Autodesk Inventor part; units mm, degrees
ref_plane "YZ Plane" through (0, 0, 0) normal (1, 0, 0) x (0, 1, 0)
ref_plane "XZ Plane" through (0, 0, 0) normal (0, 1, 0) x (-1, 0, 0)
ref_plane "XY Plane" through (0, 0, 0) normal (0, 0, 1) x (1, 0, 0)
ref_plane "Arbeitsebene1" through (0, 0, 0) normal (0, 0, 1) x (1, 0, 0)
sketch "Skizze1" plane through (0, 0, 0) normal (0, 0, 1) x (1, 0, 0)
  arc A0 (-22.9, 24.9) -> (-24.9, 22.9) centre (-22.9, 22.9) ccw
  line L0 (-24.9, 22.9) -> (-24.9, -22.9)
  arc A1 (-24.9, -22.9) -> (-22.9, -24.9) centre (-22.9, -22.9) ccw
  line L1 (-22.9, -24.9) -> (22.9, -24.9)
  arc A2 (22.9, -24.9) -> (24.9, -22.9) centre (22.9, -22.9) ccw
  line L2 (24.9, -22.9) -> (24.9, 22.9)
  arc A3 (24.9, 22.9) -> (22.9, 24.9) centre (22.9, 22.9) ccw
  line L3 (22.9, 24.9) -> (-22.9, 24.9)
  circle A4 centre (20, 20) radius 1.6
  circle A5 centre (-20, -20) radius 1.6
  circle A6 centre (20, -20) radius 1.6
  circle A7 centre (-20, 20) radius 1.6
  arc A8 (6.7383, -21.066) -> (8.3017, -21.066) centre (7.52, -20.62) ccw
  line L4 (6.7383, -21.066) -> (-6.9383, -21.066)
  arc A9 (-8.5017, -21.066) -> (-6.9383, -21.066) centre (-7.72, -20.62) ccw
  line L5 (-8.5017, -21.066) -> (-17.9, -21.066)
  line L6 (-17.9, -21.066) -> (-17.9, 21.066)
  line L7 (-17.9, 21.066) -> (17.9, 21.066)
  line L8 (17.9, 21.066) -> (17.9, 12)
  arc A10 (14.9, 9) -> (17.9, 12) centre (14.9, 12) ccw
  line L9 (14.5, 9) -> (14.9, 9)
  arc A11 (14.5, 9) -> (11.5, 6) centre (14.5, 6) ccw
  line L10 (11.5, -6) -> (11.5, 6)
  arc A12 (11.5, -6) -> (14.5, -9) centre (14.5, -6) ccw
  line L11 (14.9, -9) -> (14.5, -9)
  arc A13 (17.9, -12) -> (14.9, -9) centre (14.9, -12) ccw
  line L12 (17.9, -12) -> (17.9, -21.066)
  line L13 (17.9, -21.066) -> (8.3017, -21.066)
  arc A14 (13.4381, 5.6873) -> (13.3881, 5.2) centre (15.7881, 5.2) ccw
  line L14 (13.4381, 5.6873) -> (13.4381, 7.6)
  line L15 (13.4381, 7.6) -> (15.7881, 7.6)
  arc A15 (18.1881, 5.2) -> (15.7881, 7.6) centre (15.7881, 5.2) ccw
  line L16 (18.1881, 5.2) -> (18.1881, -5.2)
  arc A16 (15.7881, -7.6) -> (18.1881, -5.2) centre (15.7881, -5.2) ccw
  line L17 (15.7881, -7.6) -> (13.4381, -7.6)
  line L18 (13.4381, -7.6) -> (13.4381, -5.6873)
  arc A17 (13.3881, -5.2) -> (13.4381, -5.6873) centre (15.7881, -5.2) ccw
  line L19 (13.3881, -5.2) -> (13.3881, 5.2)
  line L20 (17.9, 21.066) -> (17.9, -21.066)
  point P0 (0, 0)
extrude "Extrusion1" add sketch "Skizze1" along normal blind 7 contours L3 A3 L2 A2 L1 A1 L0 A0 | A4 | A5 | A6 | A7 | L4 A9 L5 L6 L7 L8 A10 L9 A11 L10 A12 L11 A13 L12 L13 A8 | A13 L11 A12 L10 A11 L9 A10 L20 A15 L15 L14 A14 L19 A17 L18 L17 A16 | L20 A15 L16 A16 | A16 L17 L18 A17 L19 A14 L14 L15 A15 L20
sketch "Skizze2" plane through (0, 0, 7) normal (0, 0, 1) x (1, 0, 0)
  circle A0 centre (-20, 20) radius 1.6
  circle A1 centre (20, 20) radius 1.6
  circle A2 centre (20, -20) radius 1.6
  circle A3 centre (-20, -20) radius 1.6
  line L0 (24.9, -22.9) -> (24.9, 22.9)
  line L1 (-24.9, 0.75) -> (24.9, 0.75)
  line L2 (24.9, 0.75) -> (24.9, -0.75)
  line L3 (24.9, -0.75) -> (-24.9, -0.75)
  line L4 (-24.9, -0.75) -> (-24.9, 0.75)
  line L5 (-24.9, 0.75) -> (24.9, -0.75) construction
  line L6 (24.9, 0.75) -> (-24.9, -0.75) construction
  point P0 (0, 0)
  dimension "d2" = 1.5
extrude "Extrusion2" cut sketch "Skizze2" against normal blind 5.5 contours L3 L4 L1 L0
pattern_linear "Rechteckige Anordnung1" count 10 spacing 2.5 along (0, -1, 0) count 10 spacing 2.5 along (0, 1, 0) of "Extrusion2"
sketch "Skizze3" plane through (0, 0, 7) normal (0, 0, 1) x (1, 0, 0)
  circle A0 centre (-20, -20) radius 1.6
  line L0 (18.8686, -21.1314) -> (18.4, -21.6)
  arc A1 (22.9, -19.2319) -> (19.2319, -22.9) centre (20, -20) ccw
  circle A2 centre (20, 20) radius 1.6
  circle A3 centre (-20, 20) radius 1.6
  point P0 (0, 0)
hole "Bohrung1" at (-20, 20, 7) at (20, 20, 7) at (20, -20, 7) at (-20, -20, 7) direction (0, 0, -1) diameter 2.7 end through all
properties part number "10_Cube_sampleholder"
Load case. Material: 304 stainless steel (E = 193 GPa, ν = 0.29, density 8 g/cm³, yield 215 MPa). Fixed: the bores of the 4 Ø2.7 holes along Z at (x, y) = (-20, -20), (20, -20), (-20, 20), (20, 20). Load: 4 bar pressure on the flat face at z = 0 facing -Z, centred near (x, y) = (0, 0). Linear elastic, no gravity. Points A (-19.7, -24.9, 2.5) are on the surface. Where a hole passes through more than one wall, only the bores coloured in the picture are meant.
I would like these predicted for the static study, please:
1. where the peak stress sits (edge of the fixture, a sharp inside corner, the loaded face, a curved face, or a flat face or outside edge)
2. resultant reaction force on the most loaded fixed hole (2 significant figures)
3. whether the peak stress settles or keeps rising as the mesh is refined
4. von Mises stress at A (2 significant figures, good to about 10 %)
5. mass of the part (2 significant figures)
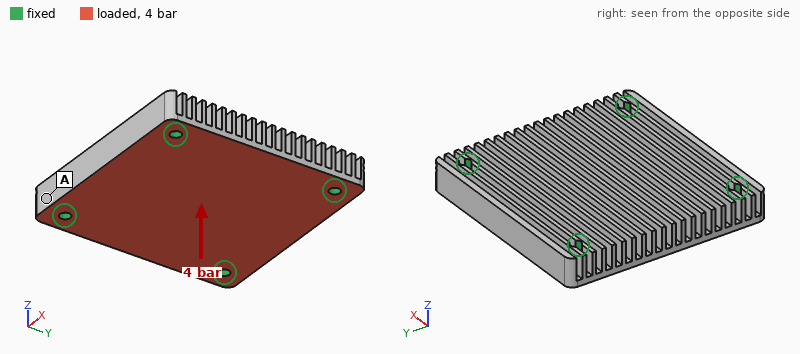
edge of the fixture
250 N
keeps rising
10 MPa
76 g
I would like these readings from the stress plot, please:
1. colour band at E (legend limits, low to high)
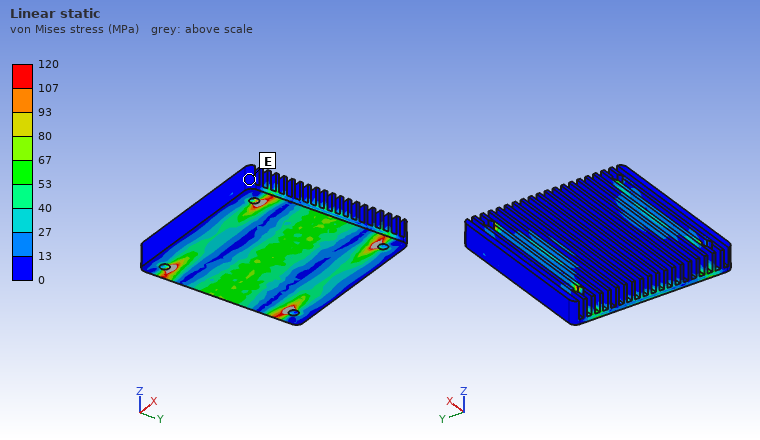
0 to 13 MPa
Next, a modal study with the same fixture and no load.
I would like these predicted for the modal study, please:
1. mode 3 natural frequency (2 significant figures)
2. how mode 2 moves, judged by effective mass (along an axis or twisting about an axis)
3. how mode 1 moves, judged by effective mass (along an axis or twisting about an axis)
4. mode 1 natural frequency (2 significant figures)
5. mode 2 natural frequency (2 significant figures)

7500 Hz
twisting about Y
along Z
3000 Hz
3900 Hz
